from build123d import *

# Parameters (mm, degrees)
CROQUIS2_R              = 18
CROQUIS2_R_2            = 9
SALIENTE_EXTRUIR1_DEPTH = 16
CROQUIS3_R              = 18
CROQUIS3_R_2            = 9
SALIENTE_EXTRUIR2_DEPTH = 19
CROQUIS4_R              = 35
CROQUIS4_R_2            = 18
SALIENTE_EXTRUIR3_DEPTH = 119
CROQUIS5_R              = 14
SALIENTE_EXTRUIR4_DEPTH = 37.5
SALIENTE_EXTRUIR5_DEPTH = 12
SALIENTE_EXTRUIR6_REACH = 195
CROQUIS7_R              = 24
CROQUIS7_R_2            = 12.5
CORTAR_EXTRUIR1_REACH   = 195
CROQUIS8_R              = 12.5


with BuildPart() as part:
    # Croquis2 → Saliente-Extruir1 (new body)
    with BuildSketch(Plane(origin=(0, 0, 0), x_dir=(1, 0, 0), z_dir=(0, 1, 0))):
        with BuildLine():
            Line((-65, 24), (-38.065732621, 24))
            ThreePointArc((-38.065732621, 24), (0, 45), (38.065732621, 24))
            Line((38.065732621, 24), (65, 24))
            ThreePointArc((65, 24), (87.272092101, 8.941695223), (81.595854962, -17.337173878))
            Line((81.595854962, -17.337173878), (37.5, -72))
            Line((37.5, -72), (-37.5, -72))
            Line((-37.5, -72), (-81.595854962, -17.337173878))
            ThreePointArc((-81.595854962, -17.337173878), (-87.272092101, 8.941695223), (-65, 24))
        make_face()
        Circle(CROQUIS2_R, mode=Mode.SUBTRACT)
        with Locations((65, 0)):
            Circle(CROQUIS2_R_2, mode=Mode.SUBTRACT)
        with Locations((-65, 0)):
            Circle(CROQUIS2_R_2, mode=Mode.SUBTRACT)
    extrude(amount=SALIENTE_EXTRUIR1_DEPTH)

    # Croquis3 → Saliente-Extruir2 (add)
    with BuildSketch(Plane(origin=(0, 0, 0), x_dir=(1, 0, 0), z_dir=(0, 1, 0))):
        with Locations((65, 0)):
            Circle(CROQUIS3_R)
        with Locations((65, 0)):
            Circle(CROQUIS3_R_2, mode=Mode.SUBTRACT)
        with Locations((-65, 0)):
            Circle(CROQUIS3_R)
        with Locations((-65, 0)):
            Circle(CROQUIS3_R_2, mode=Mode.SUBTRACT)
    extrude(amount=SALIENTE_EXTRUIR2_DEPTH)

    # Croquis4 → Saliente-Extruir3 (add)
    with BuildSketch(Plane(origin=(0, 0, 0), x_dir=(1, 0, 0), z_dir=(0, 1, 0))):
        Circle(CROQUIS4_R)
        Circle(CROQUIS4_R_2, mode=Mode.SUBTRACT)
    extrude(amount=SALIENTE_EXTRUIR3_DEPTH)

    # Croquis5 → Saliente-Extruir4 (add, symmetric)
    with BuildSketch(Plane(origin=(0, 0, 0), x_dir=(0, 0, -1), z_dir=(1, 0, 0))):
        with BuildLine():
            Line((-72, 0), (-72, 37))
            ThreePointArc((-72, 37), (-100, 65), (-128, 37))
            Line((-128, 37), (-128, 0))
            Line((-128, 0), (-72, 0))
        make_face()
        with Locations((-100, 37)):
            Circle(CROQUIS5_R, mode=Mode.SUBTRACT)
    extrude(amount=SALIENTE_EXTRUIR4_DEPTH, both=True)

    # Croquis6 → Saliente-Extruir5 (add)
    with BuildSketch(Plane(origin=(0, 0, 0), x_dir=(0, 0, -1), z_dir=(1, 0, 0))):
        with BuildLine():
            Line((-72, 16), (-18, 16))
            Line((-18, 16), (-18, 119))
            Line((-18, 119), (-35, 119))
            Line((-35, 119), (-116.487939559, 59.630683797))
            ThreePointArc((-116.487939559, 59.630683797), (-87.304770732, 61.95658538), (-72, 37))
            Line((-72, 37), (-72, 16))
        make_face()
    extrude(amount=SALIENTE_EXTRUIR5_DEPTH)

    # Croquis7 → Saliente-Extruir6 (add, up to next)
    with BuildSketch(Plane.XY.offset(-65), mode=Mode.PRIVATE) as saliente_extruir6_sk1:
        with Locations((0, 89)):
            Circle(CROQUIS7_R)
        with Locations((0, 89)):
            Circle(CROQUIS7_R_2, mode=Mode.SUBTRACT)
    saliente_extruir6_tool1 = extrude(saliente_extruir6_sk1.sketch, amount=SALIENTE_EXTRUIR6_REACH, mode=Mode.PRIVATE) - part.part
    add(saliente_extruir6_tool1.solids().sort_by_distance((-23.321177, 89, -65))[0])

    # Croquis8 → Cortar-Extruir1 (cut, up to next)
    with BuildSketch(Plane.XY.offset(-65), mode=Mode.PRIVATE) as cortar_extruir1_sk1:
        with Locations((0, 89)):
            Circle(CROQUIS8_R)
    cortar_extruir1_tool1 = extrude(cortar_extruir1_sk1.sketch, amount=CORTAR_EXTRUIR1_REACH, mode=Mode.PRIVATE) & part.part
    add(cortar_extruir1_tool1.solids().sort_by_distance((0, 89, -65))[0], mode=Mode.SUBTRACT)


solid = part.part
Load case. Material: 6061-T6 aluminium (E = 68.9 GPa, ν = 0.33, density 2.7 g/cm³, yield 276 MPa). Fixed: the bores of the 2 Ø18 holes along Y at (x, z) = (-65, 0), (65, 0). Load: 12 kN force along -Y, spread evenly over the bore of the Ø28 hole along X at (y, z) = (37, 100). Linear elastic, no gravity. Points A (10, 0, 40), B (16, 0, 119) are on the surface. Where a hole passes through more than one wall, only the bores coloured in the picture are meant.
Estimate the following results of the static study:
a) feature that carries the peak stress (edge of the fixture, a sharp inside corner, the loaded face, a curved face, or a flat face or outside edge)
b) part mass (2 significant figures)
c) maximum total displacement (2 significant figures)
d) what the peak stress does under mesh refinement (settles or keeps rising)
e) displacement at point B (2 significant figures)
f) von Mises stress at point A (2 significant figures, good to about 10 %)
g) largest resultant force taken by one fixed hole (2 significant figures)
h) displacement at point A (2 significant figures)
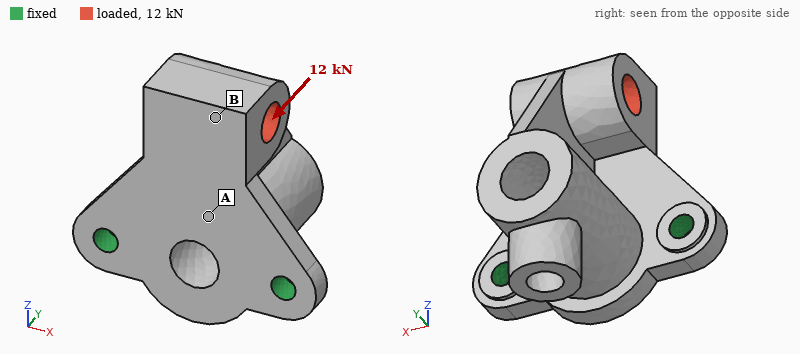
edge of the fixture
2.1 kg
0.95 mm
keeps rising
0.85 mm
45 MPa
6.2 kN
0.29 mm
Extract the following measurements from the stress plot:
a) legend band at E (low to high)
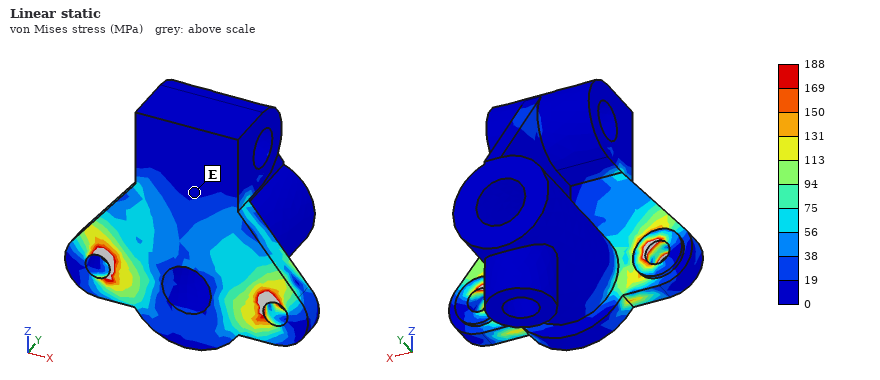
0 to 19 MPa
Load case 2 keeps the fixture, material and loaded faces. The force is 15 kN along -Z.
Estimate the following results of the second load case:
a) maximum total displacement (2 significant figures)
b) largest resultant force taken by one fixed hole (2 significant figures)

0.35 mm
8.2 kN
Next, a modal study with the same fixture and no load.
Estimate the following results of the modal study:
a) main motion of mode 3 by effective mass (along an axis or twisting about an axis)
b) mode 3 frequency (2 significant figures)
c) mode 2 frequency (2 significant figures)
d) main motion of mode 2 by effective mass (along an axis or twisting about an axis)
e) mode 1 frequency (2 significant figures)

along Y
2400 Hz
1800 Hz
along X
600 Hz
